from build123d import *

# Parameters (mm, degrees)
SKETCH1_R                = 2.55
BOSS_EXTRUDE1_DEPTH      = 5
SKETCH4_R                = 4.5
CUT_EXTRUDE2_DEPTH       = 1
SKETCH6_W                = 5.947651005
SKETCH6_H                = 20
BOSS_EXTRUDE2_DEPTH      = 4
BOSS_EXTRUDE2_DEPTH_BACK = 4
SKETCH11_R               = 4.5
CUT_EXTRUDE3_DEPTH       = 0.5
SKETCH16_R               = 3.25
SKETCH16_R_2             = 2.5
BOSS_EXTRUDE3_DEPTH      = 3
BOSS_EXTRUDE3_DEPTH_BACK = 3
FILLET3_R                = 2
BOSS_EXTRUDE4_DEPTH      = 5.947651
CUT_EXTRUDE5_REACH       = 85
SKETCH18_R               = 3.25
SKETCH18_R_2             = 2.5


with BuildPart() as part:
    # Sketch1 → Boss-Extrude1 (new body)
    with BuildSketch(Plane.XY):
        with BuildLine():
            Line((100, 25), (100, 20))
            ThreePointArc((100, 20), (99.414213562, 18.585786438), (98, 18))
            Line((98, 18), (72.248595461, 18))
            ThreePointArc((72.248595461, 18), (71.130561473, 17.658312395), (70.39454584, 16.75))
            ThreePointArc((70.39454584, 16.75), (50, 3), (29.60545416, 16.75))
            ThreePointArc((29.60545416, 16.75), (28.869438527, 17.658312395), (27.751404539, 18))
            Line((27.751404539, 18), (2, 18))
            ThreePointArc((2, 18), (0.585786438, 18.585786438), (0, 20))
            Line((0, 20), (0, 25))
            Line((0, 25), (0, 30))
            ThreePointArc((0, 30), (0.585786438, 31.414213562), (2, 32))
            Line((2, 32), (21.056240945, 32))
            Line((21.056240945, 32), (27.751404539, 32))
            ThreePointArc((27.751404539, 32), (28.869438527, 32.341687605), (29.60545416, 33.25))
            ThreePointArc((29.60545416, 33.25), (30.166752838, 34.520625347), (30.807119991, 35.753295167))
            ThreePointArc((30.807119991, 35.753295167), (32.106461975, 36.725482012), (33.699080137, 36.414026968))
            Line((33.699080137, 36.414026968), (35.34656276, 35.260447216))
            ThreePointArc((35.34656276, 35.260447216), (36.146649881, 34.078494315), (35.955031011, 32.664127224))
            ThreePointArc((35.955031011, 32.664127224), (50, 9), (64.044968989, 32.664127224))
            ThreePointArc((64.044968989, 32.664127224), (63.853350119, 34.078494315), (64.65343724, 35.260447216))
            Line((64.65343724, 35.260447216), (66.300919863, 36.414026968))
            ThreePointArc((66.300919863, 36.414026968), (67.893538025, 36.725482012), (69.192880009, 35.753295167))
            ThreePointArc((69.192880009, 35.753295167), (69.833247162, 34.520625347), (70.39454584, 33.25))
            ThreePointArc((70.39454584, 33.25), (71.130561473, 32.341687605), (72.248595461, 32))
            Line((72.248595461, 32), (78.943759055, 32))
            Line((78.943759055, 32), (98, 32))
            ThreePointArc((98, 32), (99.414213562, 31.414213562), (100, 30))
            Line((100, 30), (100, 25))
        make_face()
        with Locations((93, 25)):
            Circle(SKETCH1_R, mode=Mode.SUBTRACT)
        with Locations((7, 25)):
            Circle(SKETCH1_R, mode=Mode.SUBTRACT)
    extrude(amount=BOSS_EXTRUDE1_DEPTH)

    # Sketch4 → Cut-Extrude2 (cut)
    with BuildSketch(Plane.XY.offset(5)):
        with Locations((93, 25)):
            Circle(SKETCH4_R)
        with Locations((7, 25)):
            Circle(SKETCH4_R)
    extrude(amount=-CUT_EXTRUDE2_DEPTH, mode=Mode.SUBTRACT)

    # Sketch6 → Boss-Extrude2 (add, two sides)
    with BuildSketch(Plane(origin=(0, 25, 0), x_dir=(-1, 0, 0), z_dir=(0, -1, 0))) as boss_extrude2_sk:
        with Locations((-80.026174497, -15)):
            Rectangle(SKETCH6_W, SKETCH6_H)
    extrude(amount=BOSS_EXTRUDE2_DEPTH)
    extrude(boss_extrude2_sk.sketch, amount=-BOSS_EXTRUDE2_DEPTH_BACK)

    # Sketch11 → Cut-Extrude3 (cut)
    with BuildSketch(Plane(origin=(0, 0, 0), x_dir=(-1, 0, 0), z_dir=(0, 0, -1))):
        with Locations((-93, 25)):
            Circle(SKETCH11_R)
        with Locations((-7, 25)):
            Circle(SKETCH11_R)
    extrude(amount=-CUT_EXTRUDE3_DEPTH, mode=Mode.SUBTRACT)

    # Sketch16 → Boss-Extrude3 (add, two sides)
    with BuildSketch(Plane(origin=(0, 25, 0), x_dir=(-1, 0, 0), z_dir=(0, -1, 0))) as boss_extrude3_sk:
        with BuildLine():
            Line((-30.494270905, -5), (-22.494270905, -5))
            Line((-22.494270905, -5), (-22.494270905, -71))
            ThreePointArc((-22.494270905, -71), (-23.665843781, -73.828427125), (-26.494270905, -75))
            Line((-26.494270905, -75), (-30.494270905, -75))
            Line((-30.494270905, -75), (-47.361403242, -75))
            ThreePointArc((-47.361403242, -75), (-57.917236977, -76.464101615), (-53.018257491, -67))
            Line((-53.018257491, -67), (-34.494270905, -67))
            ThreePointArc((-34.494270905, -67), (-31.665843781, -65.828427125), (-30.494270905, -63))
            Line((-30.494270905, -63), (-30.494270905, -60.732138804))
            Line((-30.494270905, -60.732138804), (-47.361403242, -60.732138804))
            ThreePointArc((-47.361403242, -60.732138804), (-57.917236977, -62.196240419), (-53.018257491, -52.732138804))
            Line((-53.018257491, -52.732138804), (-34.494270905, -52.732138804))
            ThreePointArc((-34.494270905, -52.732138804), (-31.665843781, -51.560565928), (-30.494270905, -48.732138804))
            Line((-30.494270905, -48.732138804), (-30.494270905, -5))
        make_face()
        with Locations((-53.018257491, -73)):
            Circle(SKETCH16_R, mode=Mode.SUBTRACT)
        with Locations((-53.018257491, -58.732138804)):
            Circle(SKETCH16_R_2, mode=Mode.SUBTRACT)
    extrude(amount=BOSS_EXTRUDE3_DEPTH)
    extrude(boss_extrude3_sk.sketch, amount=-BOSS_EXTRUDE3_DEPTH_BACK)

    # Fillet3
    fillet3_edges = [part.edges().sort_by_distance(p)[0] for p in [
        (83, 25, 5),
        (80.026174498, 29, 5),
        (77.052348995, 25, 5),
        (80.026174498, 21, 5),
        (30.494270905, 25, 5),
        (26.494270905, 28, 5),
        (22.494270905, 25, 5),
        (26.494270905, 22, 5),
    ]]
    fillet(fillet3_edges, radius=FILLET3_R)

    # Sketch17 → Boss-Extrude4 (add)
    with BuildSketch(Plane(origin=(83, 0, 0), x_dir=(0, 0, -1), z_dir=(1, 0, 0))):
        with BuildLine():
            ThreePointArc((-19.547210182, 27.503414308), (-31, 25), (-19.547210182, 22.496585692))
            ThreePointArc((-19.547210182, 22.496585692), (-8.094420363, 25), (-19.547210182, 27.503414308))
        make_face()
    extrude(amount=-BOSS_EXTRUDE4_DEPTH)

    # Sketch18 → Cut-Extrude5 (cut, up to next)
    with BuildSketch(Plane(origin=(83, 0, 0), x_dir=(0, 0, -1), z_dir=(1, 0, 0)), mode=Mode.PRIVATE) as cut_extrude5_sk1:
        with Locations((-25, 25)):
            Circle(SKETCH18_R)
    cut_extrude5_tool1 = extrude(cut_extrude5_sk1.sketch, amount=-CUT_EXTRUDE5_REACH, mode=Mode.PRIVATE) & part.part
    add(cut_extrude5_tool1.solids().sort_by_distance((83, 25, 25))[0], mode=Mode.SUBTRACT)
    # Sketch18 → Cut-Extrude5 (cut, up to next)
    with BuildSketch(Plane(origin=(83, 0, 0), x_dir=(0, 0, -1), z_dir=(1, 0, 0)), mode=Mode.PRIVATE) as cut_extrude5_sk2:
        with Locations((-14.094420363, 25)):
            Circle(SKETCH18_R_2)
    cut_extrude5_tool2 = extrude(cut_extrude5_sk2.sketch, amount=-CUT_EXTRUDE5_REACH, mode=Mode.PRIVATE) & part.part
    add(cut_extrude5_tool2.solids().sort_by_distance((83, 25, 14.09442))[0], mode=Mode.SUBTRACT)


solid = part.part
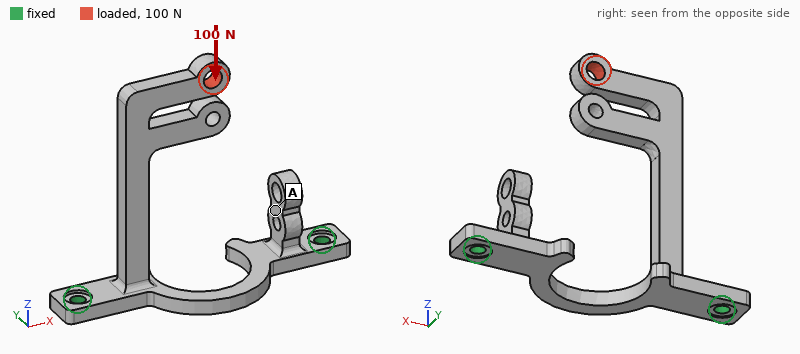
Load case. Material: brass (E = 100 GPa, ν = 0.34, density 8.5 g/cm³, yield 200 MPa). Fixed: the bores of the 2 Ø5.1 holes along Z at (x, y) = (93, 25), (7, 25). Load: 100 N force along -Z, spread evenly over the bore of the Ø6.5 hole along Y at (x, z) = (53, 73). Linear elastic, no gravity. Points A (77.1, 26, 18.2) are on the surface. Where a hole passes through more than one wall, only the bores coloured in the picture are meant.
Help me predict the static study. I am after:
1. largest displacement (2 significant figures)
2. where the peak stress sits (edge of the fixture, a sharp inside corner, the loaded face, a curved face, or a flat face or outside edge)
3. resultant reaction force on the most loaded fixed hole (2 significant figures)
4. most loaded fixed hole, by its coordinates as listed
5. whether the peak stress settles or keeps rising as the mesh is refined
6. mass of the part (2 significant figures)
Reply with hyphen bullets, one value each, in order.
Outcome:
- 0.60 mm
- edge of the fixture
- 68 N
- (7, 25)
- keeps rising
- 110 g
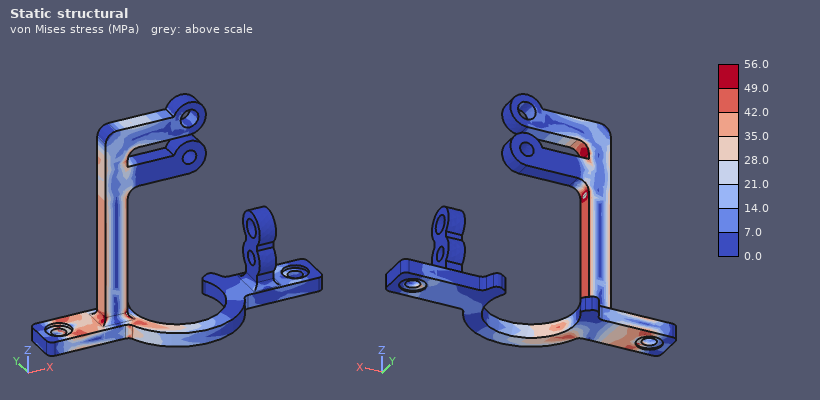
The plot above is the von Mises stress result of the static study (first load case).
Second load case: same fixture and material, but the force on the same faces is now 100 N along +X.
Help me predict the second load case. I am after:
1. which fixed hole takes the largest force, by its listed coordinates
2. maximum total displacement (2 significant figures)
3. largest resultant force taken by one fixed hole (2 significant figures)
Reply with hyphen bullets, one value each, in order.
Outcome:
- (7, 25)
- 1.0 mm
- 110 N
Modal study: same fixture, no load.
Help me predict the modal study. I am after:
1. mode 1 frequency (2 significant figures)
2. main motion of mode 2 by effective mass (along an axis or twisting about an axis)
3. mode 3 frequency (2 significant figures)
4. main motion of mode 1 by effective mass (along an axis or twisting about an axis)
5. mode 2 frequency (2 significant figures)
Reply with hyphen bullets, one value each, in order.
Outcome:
- 280 Hz
- along X
- 1200 Hz
- along Y
- 320 Hz
